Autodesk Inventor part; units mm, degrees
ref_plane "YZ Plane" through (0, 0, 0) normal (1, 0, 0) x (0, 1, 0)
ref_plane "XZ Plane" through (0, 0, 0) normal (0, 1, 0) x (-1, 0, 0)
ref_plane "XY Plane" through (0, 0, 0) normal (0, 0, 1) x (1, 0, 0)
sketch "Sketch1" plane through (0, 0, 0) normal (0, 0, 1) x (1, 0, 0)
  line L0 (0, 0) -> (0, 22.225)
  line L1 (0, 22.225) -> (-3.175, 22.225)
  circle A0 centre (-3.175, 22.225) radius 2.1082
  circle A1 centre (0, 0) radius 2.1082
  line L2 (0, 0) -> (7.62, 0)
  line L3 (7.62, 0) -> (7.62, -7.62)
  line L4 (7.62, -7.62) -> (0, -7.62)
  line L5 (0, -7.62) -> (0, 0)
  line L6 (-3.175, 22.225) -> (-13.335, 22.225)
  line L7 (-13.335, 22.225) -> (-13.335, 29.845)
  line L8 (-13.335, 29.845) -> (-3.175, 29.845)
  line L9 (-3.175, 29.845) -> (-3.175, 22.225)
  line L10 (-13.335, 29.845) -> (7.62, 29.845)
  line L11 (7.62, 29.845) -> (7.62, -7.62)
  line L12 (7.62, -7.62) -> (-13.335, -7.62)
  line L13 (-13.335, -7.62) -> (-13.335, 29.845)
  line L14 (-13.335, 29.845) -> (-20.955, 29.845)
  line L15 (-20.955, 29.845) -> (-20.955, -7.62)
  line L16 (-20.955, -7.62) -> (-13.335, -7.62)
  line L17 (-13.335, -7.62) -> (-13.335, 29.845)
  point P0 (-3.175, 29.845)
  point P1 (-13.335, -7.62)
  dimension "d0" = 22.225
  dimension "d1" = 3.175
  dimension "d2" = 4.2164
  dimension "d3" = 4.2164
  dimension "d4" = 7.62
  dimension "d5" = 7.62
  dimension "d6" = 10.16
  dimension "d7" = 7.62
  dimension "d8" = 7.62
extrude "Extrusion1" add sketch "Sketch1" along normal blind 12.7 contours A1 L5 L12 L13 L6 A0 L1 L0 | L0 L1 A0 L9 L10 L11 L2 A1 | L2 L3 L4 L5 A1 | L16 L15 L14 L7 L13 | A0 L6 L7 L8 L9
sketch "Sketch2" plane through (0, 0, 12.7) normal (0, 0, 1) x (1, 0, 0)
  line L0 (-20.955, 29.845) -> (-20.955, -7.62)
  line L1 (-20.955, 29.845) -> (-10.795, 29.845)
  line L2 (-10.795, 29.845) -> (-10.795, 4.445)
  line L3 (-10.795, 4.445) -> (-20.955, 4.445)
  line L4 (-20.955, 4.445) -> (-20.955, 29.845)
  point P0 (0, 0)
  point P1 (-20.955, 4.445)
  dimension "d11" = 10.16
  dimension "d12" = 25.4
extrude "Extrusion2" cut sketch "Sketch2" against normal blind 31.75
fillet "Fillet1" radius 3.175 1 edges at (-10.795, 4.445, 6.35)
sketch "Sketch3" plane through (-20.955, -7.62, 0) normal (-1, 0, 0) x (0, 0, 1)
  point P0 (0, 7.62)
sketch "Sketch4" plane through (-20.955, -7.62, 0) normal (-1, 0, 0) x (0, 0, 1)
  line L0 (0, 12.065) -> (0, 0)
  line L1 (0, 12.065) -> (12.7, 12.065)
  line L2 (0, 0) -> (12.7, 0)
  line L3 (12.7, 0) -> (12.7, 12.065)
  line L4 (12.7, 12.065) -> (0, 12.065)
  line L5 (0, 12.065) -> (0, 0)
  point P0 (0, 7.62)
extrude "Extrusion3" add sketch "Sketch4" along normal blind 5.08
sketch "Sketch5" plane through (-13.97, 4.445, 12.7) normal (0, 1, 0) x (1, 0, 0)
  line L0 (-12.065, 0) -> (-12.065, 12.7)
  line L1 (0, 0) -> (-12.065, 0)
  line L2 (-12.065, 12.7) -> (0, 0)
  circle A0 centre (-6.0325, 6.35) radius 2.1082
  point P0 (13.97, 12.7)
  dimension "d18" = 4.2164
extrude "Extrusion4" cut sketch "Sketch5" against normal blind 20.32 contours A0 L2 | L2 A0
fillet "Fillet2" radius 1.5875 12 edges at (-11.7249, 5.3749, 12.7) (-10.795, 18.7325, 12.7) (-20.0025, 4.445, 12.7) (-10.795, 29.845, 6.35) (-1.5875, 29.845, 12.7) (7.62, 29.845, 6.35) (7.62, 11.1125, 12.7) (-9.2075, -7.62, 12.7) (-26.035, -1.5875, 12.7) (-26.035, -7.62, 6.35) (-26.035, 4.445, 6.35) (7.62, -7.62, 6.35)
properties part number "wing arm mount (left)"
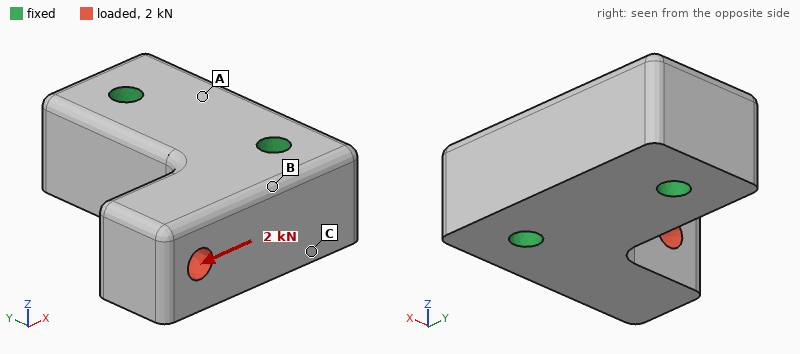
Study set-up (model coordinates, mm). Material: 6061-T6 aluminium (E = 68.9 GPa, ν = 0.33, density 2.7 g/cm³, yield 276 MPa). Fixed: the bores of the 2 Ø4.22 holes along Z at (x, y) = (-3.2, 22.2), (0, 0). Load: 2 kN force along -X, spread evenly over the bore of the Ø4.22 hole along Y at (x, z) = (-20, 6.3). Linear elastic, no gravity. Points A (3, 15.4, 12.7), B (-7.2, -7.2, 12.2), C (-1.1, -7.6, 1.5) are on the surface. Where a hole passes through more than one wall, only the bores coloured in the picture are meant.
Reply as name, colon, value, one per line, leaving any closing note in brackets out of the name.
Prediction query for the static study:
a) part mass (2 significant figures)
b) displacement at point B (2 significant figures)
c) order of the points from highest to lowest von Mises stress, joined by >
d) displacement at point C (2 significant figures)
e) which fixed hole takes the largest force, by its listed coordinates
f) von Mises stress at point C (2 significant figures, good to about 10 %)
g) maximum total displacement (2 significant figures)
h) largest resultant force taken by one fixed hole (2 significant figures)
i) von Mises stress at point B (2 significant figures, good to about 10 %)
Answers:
part mass: 28 g
displacement at point B: 2.9 µm
order of the points from highest to lowest von Mises stress, joined by >: B > C > A
displacement at point C: 1.8 µm
which fixed hole takes the largest force, by its listed coordinates: (0, 0)
von Mises stress at point C: 7.3 MPa
maximum total displacement: 7.5 µm
largest resultant force taken by one fixed hole: 2.0 kN
von Mises stress at point B: 12 MPa
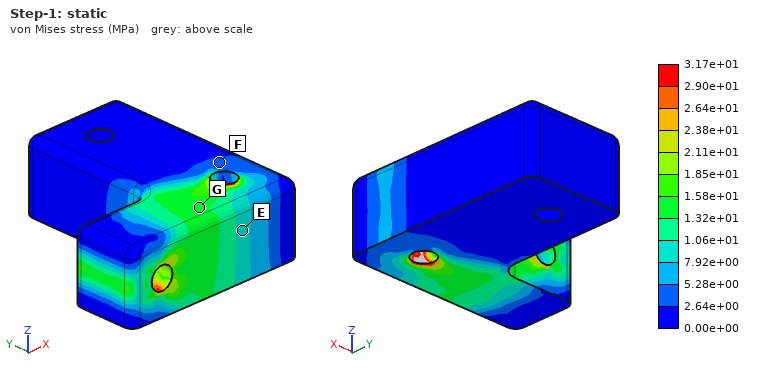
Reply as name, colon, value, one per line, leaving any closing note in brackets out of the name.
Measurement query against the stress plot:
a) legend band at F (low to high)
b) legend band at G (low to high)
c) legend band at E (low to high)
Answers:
legend band at F: 2.64e+00 to 5.28e+00 MPa
legend band at G: 1.32e+01 to 1.58e+01 MPa
legend band at E: 7.92e+00 to 1.06e+01 MPa
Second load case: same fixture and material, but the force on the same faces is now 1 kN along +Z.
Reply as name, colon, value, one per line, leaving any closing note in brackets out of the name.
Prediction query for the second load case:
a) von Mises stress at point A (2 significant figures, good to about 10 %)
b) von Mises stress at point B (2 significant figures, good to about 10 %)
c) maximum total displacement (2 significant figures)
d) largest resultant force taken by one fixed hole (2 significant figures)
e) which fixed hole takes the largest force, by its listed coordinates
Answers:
von Mises stress at point A: 5.6 MPa
von Mises stress at point B: 25 MPa
maximum total displacement: 29 µm
largest resultant force taken by one fixed hole: 920 N
which fixed hole takes the largest force, by its listed coordinates: (0, 0)
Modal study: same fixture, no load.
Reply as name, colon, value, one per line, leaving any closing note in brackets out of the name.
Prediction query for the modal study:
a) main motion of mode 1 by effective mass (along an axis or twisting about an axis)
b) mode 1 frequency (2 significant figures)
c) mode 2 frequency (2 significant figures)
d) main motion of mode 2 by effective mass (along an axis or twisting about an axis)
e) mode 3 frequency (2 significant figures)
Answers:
main motion of mode 1 by effective mass: along Z
mode 1 frequency: 15 kHz
mode 2 frequency: 18 kHz
main motion of mode 2 by effective mass: along Y
mode 3 frequency: 35 kHz
